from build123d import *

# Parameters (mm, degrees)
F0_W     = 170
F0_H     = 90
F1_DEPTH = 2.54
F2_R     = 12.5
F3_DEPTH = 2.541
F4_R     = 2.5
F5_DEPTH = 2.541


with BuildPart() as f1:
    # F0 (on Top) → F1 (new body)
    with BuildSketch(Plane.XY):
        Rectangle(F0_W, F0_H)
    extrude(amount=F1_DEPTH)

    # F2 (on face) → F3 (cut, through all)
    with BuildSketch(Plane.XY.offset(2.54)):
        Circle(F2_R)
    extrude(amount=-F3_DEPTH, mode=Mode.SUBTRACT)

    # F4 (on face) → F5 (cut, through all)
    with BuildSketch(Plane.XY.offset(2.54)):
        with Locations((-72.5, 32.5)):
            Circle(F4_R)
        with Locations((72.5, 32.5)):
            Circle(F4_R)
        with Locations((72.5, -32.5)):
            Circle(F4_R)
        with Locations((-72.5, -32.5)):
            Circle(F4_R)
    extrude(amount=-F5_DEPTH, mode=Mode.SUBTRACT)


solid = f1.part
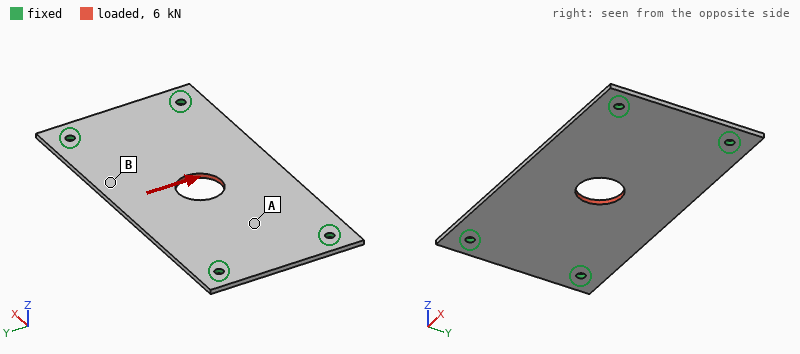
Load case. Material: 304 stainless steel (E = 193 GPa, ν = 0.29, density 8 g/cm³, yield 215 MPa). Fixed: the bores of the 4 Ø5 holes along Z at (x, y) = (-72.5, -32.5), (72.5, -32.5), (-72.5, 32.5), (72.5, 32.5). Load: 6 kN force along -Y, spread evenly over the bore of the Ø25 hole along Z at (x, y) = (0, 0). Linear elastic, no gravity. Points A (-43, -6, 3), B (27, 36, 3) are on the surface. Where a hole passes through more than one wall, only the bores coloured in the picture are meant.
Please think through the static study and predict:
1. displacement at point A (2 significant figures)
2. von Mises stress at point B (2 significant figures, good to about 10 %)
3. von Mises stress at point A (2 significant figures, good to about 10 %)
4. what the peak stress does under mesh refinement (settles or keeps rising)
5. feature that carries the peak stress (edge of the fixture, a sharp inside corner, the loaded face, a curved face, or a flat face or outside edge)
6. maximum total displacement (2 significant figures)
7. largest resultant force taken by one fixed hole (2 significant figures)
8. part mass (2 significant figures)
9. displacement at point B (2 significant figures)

8.9 µm
17 MPa
32 MPa
keeps rising
edge of the fixture
20 µm
2.1 kN
300 g
14 µm
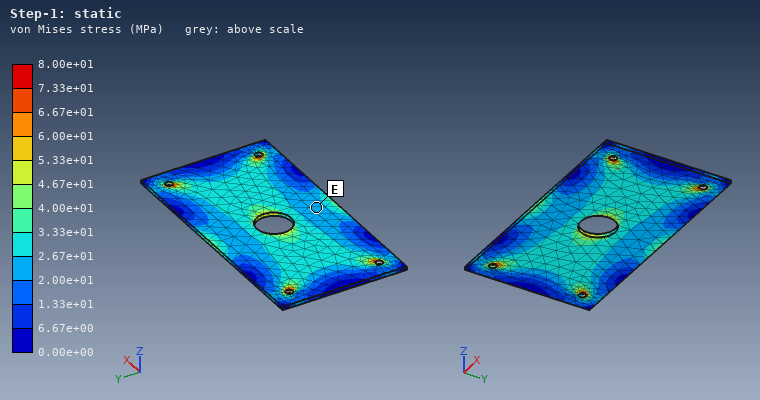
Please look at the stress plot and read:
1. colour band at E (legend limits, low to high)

2.00e+01 to 2.67e+01 MPa
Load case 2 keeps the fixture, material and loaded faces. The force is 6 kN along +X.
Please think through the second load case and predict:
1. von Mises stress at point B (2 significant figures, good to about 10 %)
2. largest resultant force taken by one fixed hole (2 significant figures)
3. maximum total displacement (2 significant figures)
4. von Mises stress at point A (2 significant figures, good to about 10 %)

8.9 MPa
1.5 kN
8.4 µm
14 MPa
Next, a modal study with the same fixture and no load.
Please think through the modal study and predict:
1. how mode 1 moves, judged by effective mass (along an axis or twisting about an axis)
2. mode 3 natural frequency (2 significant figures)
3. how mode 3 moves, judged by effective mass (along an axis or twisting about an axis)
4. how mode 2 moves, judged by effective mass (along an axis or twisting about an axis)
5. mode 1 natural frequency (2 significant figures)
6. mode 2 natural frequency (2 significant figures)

along Z
1500 Hz
twisting about Y
twisting about X
570 Hz
900 Hz
